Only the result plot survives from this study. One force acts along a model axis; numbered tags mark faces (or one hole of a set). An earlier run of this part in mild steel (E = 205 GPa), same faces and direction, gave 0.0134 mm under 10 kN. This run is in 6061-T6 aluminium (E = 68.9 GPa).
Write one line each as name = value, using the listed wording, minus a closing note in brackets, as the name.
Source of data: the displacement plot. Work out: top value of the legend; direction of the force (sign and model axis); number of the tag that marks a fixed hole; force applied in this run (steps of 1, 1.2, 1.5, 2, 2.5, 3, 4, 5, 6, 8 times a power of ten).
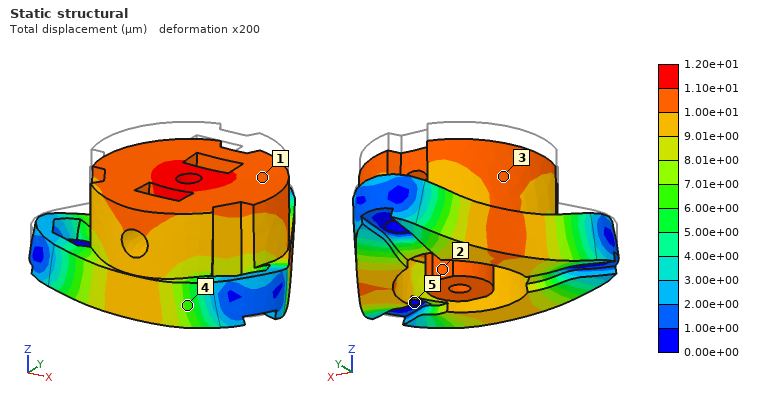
top value of the legend = 1.20e+01 µm
direction of the force = -Z
number of the tag that marks a fixed hole = 5
force applied in this run = 3 kN
